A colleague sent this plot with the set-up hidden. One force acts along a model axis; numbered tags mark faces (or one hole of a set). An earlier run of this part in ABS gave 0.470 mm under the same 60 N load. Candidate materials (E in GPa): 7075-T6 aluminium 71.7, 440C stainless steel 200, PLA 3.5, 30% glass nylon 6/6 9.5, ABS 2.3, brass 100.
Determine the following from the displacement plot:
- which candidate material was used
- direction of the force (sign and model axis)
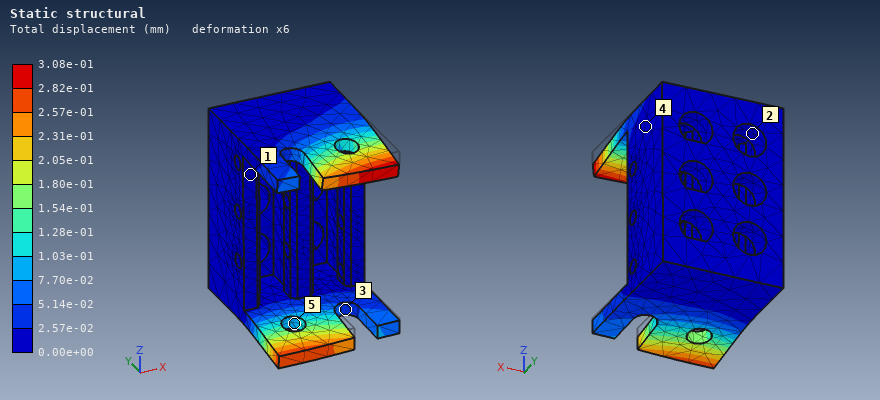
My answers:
PLA
-Z
